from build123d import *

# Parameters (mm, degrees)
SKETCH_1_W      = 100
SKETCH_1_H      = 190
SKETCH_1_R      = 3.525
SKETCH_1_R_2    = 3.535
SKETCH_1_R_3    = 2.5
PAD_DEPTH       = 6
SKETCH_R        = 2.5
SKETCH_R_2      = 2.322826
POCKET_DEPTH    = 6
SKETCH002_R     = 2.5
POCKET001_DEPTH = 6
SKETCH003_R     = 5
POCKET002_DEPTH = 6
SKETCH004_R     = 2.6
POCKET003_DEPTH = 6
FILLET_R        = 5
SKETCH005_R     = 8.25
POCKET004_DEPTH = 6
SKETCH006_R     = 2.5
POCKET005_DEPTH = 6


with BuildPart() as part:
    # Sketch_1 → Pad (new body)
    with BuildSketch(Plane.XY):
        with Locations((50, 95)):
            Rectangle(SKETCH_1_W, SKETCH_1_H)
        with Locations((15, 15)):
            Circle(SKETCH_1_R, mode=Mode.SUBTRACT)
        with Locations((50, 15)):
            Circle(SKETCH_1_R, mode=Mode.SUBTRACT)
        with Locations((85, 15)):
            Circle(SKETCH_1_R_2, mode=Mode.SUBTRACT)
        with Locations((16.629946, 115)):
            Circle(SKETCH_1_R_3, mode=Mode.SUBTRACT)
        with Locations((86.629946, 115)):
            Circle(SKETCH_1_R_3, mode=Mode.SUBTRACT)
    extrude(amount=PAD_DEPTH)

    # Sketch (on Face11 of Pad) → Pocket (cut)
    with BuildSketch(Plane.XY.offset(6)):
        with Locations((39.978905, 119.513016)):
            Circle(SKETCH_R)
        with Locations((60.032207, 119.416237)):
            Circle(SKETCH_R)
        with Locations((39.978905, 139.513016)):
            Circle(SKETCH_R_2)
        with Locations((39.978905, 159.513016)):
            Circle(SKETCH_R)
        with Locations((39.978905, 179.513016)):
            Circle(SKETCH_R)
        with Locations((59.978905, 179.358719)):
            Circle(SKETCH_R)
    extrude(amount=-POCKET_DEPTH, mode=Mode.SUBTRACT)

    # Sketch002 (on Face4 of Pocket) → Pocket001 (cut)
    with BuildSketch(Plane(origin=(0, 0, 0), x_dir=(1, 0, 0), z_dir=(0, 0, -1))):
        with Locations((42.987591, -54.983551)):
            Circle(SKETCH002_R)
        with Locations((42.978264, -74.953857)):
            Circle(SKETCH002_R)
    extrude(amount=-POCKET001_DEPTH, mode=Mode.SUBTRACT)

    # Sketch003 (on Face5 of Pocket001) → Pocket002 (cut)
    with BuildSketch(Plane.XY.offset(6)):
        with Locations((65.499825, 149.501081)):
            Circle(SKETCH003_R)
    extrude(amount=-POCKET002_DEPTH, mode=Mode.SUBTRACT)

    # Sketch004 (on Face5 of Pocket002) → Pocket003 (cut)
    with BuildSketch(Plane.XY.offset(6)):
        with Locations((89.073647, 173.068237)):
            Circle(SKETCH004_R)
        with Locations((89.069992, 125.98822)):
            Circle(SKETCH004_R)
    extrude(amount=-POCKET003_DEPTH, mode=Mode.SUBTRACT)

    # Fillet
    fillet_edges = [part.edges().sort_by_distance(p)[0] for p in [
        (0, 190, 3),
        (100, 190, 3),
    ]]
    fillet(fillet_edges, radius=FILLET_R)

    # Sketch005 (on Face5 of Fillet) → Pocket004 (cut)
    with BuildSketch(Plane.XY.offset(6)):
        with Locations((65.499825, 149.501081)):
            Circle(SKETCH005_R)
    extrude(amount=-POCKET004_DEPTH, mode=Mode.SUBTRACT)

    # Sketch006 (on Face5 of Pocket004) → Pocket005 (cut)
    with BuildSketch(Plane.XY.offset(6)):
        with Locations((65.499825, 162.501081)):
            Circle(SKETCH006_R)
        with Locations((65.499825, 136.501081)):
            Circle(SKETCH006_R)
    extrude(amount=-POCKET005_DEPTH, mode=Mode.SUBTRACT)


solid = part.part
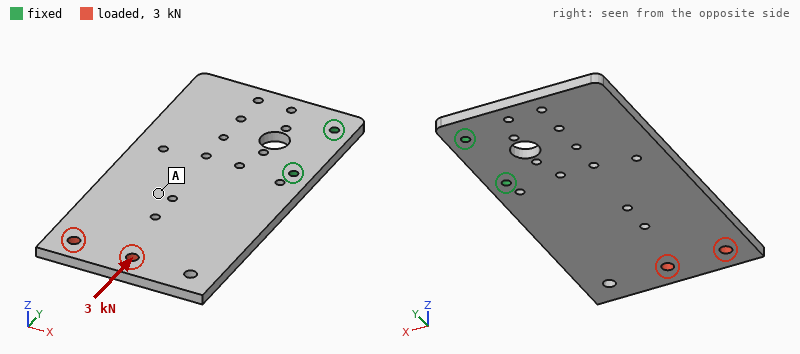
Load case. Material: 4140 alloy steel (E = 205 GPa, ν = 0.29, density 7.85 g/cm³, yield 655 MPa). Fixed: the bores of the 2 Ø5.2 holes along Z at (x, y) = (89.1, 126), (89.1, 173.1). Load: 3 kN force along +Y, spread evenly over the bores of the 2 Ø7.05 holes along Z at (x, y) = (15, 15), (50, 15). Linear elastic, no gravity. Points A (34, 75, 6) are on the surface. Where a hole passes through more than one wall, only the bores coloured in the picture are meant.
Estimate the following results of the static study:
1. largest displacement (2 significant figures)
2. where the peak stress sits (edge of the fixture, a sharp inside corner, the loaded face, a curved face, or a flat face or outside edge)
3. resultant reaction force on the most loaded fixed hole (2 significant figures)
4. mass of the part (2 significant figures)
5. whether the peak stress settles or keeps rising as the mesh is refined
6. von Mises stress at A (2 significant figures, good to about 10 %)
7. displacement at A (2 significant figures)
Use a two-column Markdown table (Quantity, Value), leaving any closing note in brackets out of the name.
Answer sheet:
| Quantity | Value |
|---|---|
| largest displacement | 46 µm |
| where the peak stress sits | edge of the fixture |
| resultant reaction force on the most loaded fixed hole | 3.7 kN |
| mass of the part | 870 g |
| whether the peak stress settles or keeps rising as the mesh is refined | keeps rising |
| von Mises stress at A | 6.2 MPa |
| displacement at A | 22 µm |
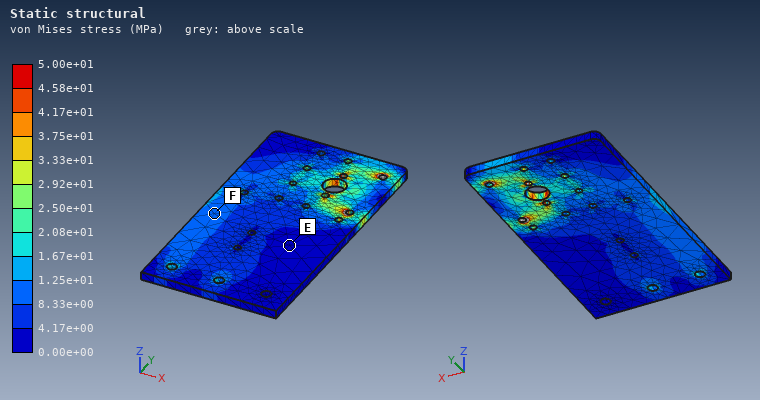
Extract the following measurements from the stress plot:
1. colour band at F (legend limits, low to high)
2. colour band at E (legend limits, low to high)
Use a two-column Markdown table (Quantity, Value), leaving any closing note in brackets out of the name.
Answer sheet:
| Quantity | Value |
|---|---|
| colour band at F | 8.33e+00 to 1.25e+01 MPa |
| colour band at E | 0.00e+00 to 4.17e+00 MPa |
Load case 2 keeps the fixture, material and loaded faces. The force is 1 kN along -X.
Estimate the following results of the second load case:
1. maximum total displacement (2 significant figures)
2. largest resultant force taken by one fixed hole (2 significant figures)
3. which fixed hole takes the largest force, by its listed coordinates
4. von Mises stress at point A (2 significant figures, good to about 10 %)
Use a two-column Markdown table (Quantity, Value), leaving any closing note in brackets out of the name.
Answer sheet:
| Quantity | Value |
|---|---|
| maximum total displacement | 38 µm |
| largest resultant force taken by one fixed hole | 3.2 kN |
| which fixed hole takes the largest force, by its listed coordinates | (89.1, 126) |
| von Mises stress at point A | 4.9 MPa |
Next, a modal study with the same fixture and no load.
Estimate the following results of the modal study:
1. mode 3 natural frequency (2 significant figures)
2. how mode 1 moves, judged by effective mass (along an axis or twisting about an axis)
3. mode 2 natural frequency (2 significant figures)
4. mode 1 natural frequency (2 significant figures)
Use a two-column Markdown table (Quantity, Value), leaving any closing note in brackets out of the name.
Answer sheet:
| Quantity | Value |
|---|---|
| mode 3 natural frequency | 950 Hz |
| how mode 1 moves, judged by effective mass | along Z |
| mode 2 natural frequency | 470 Hz |
| mode 1 natural frequency | 230 Hz |
